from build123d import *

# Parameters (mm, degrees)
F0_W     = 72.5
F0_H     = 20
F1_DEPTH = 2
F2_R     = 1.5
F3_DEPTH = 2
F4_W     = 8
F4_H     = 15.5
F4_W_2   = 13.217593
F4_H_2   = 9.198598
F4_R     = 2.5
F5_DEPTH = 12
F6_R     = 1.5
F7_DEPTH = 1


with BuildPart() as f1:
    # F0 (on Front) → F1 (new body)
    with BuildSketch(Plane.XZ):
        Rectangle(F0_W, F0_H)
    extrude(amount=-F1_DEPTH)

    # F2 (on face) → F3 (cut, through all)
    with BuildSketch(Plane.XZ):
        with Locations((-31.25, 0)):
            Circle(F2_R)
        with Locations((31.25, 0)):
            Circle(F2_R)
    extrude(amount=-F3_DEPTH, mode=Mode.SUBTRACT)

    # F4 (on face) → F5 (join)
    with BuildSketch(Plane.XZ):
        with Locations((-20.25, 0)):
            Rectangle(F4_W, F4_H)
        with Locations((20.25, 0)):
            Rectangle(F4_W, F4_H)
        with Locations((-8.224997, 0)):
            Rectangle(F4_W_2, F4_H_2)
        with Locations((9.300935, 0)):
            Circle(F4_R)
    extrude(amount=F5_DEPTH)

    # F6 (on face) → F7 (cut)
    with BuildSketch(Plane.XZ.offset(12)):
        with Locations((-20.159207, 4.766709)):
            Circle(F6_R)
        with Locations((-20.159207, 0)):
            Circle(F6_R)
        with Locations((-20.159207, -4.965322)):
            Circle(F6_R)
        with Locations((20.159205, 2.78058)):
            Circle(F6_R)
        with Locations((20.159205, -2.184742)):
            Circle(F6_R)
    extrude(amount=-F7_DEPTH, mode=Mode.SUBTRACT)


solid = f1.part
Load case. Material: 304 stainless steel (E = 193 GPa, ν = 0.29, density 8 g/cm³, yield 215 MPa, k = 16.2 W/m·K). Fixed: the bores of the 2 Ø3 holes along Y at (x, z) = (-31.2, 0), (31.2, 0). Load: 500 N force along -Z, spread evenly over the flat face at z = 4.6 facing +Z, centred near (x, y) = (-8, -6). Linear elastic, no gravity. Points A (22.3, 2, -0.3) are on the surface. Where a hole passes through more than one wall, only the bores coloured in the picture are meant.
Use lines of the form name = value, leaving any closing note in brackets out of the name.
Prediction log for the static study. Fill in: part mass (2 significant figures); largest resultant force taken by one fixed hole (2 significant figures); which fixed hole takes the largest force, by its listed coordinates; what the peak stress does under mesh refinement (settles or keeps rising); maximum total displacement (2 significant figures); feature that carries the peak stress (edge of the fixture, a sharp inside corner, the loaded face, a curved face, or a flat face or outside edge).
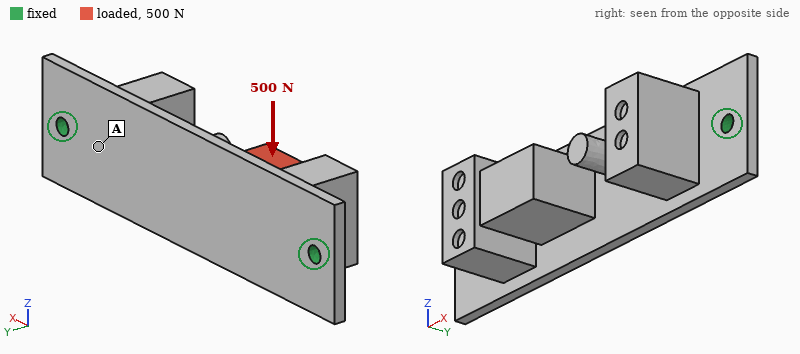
part mass = 60 g
largest resultant force taken by one fixed hole = 320 N
which fixed hole takes the largest force, by its listed coordinates = (-31.2, 0)
what the peak stress does under mesh refinement = keeps rising
maximum total displacement = 72 µm
feature that carries the peak stress = edge of the fixture
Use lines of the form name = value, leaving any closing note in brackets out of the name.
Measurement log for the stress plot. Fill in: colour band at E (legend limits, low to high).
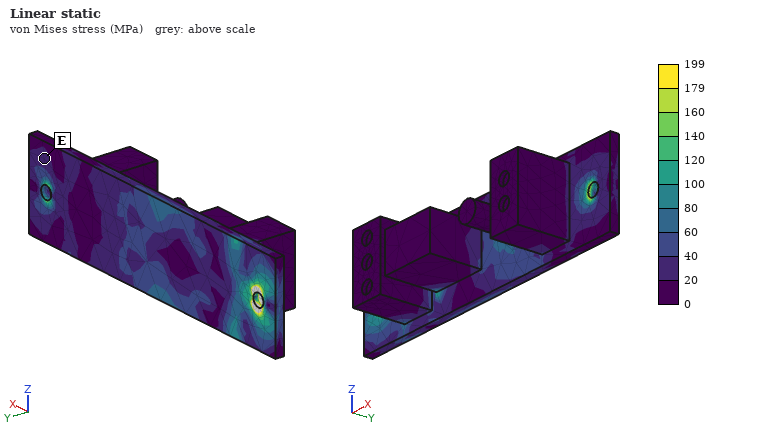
colour band at E = 20 to 40 MPa
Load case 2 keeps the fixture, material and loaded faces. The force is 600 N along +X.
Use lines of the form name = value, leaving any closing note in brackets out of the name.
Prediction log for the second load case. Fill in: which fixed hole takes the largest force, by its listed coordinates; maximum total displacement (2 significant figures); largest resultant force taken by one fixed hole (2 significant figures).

which fixed hole takes the largest force, by its listed coordinates = (-31.2, 0)
maximum total displacement = 71 µm
largest resultant force taken by one fixed hole = 410 N
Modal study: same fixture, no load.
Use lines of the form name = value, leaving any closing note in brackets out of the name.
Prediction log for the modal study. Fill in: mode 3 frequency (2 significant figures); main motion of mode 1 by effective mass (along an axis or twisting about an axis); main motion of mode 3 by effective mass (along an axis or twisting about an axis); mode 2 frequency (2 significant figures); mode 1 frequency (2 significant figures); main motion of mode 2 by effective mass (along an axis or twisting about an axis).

mode 3 frequency = 4300 Hz
main motion of mode 1 by effective mass = along Y
main motion of mode 3 by effective mass = twisting about Z
mode 2 frequency = 2900 Hz
mode 1 frequency = 1600 Hz
main motion of mode 2 by effective mass = along Z
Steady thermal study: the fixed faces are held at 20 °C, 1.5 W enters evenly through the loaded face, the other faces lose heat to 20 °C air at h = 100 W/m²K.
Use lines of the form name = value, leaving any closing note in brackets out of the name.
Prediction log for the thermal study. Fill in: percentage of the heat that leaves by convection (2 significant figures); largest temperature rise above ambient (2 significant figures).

percentage of the heat that leaves by convection = 90 %
largest temperature rise above ambient = 12 K
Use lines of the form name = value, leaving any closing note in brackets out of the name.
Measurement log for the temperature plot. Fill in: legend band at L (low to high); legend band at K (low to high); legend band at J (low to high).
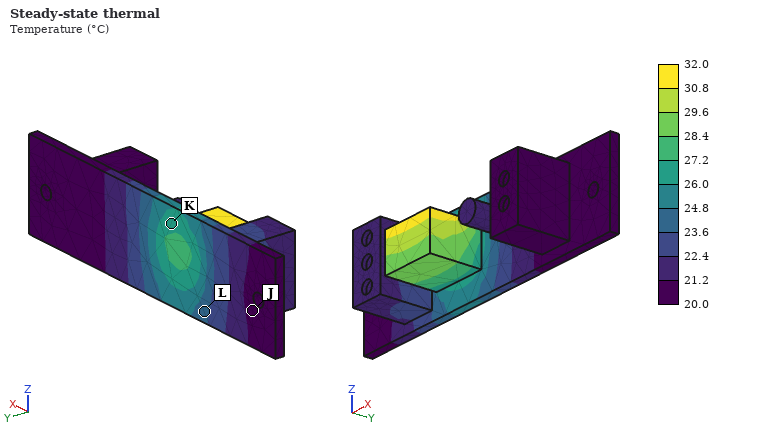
legend band at L = 23.6 to 24.8 °C
legend band at K = 26.0 to 27.2 °C
legend band at J = 20.0 to 21.2 °C
